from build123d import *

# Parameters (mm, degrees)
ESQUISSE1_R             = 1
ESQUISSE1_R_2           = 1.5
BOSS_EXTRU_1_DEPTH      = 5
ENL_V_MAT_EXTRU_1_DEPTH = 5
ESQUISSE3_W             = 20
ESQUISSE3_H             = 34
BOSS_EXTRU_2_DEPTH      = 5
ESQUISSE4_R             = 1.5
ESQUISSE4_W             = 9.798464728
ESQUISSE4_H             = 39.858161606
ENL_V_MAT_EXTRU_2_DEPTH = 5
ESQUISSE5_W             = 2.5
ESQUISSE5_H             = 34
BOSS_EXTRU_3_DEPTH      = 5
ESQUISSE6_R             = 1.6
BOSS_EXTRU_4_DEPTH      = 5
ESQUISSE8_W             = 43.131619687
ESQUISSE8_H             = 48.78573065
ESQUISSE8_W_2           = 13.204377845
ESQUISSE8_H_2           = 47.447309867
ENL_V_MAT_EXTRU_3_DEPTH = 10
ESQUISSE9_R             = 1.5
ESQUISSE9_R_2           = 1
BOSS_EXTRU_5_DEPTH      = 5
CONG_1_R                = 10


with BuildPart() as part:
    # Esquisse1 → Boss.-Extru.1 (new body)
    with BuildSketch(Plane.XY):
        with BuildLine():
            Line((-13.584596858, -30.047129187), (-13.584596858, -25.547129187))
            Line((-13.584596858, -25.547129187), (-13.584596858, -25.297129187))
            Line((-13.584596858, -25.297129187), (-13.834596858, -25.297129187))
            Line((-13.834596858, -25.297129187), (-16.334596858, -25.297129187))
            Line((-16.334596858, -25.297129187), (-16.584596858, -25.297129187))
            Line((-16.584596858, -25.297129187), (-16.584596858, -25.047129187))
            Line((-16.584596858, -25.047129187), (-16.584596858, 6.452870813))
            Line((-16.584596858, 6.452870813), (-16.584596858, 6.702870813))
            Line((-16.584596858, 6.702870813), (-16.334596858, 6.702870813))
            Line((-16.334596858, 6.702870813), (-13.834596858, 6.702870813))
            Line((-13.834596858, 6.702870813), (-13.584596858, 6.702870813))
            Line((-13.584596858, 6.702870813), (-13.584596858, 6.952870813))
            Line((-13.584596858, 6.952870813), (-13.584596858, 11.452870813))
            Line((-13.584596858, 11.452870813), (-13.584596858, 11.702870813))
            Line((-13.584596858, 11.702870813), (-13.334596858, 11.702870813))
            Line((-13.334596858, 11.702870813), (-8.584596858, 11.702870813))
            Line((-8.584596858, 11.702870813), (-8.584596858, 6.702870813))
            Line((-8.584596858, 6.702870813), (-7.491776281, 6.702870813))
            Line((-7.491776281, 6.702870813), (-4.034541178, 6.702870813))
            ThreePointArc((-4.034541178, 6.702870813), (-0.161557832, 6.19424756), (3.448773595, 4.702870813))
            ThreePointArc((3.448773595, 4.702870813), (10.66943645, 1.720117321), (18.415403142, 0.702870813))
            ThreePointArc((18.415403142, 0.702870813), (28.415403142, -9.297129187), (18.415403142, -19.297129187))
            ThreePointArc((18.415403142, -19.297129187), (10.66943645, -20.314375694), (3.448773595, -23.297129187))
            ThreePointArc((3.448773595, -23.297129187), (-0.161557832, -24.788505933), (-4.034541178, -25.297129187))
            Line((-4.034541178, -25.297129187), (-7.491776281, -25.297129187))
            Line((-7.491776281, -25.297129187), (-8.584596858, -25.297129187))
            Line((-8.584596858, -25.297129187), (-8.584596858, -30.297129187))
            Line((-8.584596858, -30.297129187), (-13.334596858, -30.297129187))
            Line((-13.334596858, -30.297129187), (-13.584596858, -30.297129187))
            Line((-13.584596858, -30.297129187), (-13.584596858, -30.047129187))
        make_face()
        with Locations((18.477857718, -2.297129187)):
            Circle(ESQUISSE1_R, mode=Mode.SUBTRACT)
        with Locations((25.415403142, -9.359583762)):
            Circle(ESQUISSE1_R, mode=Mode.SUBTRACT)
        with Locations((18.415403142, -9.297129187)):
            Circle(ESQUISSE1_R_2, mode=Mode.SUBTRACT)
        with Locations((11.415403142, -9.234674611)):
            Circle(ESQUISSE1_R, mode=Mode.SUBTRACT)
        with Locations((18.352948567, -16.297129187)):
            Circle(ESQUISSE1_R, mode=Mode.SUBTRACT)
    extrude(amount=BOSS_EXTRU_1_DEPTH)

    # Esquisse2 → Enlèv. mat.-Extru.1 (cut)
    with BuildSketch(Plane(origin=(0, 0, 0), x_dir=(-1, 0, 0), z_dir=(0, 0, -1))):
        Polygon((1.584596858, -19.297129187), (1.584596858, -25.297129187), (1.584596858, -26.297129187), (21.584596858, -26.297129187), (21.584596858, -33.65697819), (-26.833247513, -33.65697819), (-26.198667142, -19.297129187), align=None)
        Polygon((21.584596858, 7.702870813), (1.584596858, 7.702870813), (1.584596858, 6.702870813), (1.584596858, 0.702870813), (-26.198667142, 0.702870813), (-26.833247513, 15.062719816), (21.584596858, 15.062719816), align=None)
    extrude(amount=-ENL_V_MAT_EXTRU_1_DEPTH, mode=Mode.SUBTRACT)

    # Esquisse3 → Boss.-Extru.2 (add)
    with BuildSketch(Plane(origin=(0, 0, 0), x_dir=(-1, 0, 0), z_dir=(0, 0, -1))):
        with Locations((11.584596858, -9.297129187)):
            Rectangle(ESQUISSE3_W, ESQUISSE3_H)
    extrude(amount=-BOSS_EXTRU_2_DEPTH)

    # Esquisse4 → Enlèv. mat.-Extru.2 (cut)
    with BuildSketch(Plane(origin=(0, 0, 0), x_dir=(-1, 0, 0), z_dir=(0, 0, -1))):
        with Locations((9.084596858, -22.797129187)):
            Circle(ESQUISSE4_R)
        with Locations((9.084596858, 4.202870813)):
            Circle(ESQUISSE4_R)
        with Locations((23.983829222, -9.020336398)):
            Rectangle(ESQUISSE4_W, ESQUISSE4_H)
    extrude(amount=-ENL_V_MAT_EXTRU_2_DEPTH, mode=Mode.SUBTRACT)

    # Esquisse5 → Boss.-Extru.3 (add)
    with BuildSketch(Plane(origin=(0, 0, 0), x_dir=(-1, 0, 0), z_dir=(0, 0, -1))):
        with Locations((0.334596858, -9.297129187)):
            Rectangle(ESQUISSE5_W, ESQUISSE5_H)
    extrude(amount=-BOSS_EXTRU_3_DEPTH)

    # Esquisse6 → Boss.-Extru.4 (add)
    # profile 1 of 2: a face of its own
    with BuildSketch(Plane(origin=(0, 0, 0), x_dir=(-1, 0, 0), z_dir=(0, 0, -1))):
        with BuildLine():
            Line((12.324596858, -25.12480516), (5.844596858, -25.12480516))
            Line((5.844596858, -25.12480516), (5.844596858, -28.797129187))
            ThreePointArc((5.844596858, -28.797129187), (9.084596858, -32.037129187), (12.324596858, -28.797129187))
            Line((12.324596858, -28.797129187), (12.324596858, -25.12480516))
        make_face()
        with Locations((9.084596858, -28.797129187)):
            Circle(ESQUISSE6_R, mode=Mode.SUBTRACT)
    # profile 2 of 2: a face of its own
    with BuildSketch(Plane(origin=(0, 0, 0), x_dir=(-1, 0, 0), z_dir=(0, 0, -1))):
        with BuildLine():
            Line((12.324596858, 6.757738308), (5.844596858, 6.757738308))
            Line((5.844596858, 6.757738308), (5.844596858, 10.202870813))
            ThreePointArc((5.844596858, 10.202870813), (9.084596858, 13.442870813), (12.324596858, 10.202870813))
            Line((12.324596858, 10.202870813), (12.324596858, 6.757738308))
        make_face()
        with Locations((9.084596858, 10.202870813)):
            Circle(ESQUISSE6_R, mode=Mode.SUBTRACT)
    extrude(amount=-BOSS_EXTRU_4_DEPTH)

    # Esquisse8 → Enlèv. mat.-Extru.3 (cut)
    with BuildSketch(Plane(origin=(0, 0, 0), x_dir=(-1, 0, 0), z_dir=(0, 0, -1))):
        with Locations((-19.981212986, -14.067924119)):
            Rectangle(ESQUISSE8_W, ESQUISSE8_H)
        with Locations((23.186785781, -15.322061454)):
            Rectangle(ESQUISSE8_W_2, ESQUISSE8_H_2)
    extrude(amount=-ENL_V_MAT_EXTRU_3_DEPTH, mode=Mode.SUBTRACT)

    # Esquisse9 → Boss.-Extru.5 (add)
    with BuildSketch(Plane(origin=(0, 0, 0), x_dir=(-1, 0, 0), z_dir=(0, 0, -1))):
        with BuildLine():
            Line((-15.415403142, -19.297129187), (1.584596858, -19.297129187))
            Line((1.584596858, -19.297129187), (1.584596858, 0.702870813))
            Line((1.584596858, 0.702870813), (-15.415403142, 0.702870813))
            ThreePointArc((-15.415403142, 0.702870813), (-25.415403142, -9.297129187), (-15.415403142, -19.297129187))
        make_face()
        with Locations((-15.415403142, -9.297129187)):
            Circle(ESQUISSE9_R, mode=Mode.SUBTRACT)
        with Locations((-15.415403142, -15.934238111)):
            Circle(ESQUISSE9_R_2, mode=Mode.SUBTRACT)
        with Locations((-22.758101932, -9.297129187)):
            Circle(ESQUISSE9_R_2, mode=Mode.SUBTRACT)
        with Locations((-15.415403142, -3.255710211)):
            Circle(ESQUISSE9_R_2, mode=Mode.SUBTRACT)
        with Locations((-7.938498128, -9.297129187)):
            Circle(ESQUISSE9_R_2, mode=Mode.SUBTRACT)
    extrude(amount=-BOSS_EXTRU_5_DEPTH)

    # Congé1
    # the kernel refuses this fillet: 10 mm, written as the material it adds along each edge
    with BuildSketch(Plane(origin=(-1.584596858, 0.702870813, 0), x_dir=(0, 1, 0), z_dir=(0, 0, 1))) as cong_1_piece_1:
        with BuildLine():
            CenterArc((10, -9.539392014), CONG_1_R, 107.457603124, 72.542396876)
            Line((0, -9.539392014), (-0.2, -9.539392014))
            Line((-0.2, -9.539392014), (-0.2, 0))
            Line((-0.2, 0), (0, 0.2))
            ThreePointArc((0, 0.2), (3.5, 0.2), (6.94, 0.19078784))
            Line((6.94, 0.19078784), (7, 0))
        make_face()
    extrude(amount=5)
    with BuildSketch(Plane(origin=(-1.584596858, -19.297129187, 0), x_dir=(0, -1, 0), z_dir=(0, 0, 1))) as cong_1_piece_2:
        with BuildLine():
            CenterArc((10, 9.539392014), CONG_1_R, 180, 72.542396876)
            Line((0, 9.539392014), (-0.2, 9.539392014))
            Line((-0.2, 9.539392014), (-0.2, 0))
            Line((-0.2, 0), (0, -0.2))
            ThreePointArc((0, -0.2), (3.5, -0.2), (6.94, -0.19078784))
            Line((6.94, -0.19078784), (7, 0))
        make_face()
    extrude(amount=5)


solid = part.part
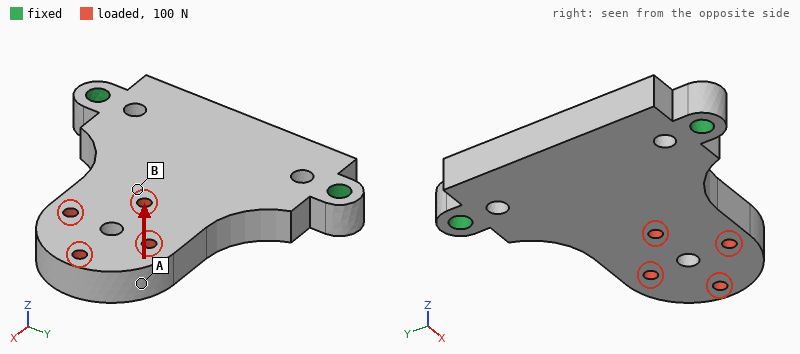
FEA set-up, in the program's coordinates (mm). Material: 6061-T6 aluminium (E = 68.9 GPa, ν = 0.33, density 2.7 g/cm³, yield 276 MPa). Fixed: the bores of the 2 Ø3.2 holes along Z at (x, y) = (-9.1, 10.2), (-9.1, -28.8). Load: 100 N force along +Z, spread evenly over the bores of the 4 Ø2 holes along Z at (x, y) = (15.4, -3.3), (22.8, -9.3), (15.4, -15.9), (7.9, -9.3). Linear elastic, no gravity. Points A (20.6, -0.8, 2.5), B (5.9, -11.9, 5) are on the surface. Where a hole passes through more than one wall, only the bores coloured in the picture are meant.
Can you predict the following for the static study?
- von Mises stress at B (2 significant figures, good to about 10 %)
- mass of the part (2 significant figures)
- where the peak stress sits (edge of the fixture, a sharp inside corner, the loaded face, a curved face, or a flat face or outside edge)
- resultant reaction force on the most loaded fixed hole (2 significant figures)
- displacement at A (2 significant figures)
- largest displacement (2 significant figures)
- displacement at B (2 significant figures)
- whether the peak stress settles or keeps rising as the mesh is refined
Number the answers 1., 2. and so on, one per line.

1. 13 MPa
2. 14 g
3. edge of the fixture
4. 50 N
5. 76 µm
6. 92 µm
7. 34 µm
8. keeps rising
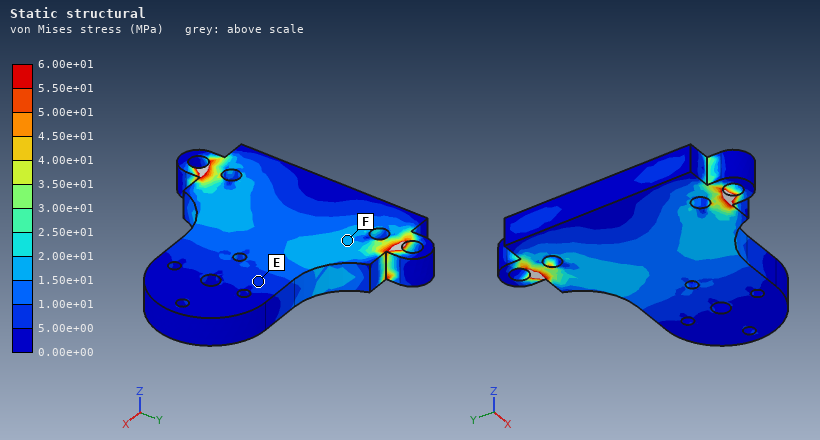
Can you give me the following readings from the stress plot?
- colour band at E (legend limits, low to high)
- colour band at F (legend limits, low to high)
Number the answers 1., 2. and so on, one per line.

1. 5.00e+00 to 1.00e+01 MPa
2. 1.50e+01 to 2.00e+01 MPa
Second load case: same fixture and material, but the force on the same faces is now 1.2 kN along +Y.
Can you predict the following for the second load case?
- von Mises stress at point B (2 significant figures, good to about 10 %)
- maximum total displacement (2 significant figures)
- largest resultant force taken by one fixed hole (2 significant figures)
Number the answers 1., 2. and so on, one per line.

1. 19 MPa
2. 36 µm
3. 1.0 kN
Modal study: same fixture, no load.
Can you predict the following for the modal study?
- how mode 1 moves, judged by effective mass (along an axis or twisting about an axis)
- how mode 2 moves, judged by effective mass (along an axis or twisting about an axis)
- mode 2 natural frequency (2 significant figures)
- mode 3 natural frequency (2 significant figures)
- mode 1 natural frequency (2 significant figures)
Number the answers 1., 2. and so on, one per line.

1. along Z
2. along Z
3. 13 kHz
4. 14 kHz
5. 2900 Hz
